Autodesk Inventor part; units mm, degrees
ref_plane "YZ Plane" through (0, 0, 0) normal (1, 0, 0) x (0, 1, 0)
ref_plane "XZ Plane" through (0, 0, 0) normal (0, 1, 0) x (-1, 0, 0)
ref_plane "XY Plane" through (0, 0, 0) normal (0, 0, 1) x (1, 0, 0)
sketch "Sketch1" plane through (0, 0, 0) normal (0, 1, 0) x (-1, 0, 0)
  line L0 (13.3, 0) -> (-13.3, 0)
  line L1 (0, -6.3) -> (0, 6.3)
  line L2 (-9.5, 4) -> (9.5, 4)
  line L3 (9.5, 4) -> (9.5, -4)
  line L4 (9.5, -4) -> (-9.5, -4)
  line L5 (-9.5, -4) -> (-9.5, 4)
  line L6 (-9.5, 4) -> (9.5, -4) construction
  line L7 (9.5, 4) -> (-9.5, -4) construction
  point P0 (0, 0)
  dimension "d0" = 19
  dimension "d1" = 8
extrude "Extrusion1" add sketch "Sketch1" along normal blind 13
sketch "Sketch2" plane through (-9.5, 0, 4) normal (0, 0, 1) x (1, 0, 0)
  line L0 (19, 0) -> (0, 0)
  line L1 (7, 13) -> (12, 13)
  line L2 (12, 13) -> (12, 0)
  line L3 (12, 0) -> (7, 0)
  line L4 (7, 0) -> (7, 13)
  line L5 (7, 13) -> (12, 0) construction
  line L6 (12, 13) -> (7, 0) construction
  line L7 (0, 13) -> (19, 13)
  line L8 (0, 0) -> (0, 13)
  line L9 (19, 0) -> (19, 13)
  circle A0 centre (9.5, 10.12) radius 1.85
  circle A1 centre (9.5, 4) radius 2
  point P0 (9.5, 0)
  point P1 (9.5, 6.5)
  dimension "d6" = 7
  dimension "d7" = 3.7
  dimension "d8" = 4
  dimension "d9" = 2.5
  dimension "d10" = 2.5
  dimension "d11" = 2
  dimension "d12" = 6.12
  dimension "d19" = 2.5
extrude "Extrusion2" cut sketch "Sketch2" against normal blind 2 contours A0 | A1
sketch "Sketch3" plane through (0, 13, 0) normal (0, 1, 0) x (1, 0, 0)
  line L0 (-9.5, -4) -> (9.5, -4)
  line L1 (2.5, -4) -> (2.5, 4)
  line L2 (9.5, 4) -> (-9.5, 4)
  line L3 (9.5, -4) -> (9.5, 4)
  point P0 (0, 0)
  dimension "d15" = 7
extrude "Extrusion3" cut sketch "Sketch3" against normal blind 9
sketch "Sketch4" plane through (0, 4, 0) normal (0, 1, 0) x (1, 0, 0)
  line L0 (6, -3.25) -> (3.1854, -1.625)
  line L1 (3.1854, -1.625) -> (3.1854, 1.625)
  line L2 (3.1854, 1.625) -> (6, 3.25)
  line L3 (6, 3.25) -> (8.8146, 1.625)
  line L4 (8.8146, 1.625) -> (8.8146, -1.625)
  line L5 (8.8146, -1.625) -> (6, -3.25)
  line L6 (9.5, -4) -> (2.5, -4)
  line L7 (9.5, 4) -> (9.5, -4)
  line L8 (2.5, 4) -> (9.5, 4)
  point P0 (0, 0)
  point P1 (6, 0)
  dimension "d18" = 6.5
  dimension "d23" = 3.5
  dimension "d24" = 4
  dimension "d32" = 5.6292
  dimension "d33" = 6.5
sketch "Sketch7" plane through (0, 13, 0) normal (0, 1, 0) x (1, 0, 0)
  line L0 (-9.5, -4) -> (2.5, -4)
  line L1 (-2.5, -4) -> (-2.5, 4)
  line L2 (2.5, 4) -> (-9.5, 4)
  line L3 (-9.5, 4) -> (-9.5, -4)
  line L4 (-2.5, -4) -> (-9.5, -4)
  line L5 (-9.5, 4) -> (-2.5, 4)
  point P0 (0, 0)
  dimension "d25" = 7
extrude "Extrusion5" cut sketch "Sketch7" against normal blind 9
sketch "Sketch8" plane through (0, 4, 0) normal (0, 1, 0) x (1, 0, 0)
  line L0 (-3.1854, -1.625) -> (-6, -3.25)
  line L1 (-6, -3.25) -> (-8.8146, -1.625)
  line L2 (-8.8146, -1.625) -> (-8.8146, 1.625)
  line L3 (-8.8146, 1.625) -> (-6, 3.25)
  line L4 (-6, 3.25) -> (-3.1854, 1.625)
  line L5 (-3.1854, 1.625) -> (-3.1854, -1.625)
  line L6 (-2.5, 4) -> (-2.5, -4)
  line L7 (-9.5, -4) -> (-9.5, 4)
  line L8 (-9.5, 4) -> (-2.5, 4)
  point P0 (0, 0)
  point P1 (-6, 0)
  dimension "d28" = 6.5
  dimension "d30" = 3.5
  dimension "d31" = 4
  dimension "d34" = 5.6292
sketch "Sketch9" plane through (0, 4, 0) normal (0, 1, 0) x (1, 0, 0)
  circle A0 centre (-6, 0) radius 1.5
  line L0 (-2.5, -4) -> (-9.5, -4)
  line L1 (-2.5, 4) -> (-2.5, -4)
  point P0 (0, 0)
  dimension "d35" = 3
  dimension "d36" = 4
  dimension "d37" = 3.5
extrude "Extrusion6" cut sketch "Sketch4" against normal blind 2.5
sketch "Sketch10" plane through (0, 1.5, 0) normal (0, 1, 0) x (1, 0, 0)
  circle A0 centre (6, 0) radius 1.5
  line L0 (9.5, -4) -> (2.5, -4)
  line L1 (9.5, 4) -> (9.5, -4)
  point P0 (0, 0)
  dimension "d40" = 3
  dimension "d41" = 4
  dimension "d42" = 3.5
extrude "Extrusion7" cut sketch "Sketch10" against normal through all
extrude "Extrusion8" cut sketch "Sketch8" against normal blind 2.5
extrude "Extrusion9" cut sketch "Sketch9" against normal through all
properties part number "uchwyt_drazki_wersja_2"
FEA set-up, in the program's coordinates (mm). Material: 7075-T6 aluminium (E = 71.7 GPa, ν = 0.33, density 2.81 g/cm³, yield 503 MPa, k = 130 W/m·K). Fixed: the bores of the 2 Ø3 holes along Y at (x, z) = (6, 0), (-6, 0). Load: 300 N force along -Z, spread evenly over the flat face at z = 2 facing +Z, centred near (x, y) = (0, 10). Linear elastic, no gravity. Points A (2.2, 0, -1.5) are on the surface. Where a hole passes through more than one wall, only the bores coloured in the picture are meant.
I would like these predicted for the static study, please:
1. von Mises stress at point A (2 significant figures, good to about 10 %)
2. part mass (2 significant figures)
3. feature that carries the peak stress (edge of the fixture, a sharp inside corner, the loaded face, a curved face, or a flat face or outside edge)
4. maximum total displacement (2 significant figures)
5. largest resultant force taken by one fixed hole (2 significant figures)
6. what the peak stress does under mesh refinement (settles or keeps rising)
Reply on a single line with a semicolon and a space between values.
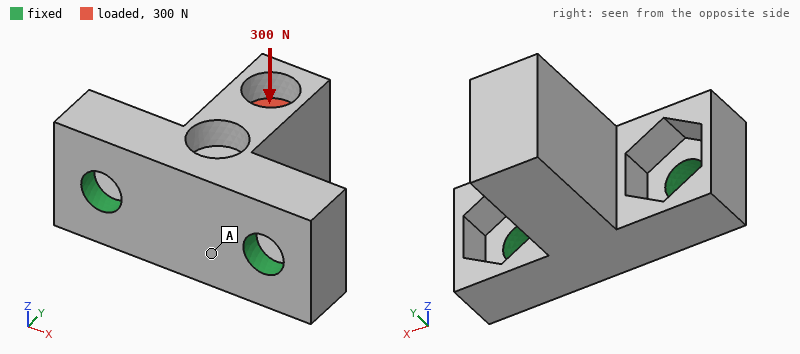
42 MPa; 2.1 g; edge of the fixture; 67 µm; 150 N; keeps rising
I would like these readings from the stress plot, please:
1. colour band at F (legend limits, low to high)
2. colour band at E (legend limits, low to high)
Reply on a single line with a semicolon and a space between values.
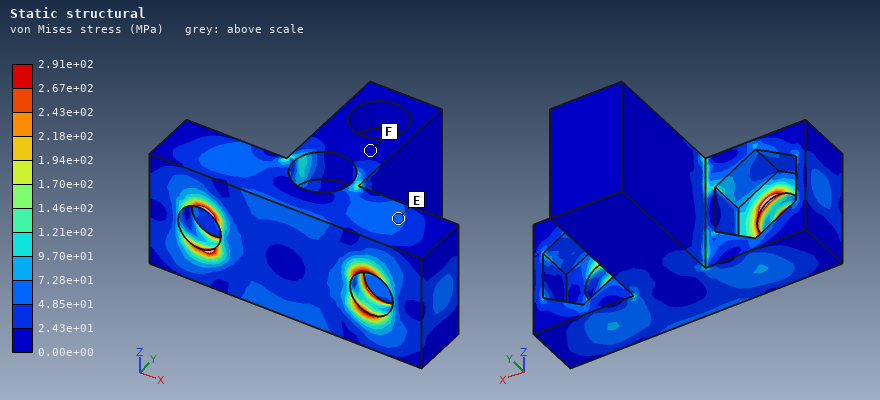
0.00e+00 to 2.43e+01 MPa; 4.85e+01 to 7.28e+01 MPa
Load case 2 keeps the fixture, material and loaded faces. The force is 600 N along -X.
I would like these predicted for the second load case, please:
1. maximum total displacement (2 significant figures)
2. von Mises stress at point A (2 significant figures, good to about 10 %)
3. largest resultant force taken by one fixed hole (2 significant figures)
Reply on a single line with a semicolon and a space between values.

64 µm; 64 MPa; 640 N
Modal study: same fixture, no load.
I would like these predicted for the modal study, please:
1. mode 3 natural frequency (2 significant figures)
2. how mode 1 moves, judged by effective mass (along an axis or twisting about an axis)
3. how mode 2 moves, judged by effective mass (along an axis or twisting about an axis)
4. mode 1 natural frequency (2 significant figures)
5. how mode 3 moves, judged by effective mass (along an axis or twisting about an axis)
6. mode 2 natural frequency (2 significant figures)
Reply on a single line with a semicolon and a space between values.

42 kHz; along Z; along X; 14 kHz; along Y; 25 kHz
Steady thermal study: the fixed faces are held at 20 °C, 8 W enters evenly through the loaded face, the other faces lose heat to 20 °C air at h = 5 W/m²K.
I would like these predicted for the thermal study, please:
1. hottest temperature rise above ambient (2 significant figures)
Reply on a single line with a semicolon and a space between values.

26 K
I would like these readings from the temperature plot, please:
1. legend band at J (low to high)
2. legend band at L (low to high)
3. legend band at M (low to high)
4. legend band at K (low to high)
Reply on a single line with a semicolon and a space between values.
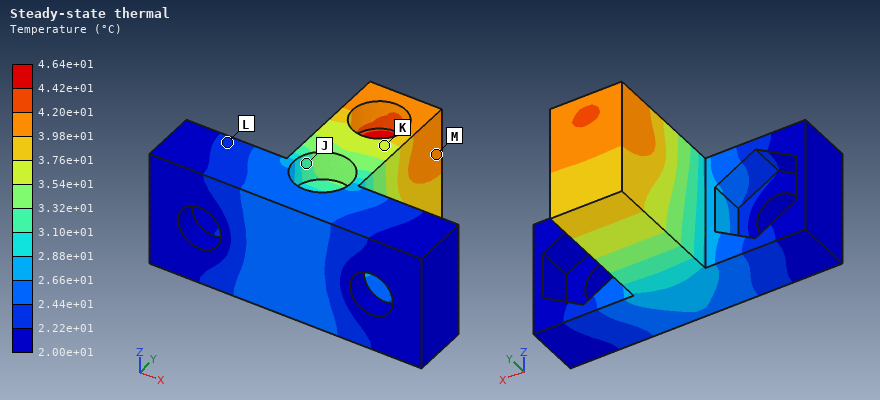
3.10e+01 to 3.32e+01 °C; 2.22e+01 to 2.44e+01 °C; 3.98e+01 to 4.20e+01 °C; 3.54e+01 to 3.76e+01 °C
